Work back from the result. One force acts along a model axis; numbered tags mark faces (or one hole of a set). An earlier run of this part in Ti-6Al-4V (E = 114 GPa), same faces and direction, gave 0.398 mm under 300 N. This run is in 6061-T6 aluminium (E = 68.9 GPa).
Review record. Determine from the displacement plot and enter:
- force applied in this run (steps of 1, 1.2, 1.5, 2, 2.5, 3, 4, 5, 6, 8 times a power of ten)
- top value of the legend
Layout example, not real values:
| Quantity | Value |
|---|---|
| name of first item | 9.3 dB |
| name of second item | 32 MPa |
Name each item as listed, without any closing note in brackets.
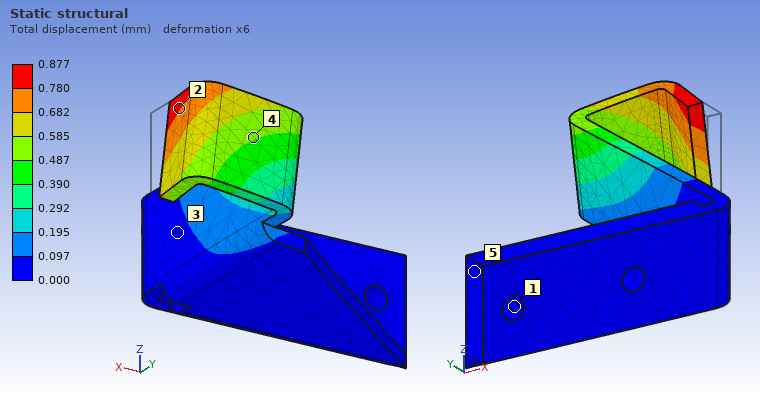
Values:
| Quantity | Value |
|---|---|
| force applied in this run | 400 N |
| top value of the legend | 0.877 mm |
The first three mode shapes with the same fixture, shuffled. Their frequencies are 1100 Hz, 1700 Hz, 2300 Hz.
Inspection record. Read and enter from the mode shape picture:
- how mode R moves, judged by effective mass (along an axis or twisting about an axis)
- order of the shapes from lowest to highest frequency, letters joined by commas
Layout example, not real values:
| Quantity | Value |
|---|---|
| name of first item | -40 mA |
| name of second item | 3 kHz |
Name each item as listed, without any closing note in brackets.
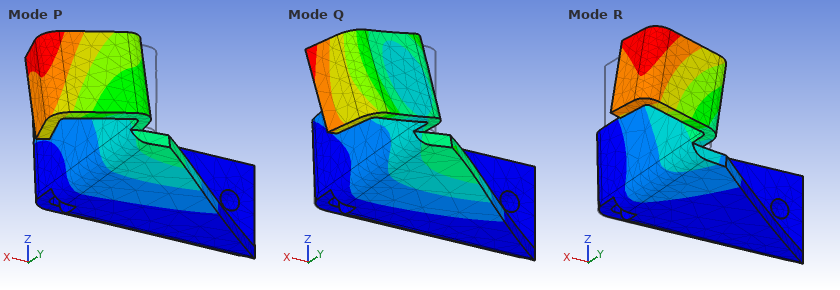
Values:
| Quantity | Value |
|---|---|
| how mode R moves, judged by effective mass | along Z |
| order of the shapes from lowest to highest frequency, letters joined by commas | R, P, Q |
